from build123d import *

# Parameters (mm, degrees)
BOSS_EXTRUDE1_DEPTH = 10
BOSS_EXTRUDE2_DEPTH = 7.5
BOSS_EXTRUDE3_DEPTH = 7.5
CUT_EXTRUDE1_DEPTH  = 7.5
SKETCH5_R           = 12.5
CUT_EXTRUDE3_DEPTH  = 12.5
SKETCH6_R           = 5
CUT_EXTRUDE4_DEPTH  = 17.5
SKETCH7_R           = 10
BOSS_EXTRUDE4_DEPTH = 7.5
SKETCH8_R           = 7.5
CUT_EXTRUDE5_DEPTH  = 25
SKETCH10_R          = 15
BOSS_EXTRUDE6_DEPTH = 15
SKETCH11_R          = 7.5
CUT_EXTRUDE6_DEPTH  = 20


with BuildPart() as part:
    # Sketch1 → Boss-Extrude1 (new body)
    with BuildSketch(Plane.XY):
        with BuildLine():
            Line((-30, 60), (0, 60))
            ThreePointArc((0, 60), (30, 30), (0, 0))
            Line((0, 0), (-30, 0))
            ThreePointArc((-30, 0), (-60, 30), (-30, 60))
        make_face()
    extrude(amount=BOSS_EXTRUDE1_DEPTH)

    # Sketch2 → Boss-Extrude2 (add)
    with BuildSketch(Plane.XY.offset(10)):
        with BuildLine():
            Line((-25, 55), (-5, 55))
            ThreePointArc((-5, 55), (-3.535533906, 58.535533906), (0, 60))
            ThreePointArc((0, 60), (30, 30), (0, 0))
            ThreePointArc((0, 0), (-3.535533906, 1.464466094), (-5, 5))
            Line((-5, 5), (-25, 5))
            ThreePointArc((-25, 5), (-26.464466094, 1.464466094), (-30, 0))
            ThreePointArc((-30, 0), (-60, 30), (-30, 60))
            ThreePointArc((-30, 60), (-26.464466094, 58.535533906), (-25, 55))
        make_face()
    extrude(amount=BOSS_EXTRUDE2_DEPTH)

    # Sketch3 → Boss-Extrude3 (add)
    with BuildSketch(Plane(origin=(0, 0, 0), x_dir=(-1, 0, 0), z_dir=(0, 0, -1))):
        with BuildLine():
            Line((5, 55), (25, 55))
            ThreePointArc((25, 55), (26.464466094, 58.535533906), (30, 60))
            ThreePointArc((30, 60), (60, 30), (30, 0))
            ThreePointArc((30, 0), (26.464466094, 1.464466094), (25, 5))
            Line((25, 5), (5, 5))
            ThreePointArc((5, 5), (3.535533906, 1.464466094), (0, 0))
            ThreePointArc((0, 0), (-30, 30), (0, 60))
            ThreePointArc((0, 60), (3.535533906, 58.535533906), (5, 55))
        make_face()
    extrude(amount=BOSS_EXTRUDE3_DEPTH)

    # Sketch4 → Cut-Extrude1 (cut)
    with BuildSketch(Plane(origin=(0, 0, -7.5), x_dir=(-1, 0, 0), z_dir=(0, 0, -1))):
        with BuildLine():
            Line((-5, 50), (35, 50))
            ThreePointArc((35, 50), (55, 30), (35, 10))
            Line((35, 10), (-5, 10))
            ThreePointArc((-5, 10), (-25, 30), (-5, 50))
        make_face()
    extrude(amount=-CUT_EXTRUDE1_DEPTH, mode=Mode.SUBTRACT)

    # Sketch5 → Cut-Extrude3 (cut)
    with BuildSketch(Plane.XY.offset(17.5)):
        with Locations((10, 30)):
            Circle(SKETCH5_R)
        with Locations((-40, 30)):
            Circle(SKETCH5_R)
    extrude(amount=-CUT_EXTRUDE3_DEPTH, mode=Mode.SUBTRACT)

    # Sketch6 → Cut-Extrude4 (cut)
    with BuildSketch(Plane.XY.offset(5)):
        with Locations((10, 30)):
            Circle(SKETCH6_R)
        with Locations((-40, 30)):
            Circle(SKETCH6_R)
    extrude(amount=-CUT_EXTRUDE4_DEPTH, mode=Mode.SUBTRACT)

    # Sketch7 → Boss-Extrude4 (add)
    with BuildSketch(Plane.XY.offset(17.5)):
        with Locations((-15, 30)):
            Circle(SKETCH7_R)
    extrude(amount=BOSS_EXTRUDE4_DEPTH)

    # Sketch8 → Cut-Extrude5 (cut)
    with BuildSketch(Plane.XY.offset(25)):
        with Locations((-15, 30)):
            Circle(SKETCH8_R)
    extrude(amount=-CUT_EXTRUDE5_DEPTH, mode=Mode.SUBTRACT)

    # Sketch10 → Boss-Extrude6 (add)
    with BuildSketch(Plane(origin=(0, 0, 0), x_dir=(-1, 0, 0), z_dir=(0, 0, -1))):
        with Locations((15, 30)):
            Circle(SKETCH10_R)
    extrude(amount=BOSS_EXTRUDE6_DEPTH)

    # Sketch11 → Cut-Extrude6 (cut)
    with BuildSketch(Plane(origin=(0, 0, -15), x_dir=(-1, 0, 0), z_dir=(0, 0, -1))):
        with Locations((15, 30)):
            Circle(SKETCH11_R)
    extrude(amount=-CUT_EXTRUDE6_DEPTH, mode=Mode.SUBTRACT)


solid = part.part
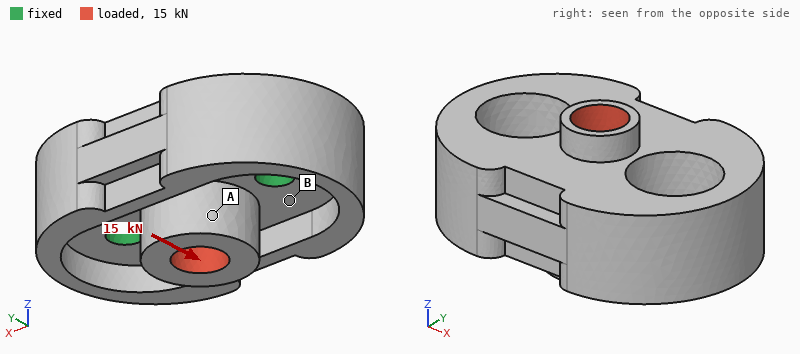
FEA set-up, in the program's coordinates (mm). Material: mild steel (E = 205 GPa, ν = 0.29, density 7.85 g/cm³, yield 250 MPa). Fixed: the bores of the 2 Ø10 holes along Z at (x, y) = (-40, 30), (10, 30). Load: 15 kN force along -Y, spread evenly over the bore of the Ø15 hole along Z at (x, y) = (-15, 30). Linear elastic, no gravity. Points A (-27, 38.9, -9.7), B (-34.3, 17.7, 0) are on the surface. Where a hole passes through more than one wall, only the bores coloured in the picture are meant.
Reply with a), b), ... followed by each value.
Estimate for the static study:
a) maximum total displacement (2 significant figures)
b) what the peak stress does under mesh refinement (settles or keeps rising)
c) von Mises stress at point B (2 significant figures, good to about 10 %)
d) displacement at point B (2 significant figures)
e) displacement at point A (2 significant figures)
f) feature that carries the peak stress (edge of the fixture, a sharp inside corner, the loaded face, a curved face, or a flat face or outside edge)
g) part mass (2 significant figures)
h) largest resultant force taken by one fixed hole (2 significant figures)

a) 20 µm
b) keeps rising
c) 46 MPa
d) 4.6 µm
e) 3.4 µm
f) edge of the fixture
g) 660 g
h) 7.5 kN
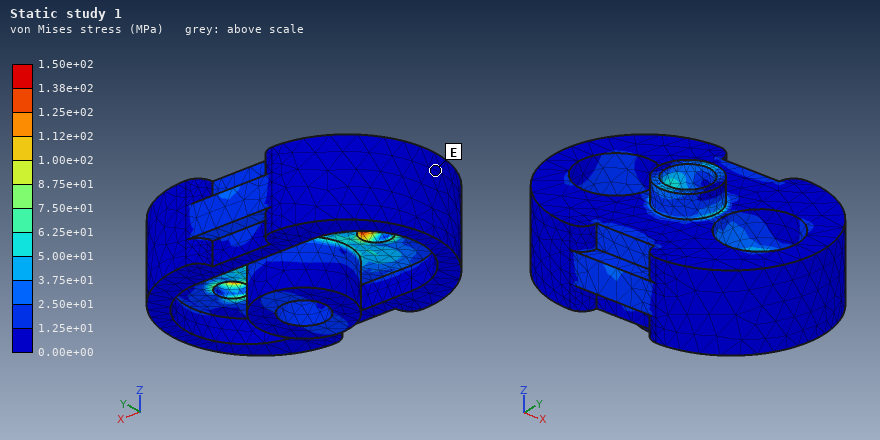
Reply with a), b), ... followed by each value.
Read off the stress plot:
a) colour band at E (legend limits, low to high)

a) 0.00e+00 to 1.25e+01 MPa
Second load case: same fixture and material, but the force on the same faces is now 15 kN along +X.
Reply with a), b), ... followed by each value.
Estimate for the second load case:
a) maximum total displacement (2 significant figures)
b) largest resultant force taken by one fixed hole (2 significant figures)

a) 9.2 µm
b) 7.5 kN
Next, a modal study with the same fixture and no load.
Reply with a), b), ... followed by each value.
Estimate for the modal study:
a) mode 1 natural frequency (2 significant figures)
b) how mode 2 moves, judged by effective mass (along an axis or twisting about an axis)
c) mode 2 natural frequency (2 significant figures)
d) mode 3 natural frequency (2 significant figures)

a) 3200 Hz
b) along Z
c) 8000 Hz
d) 8900 Hz
